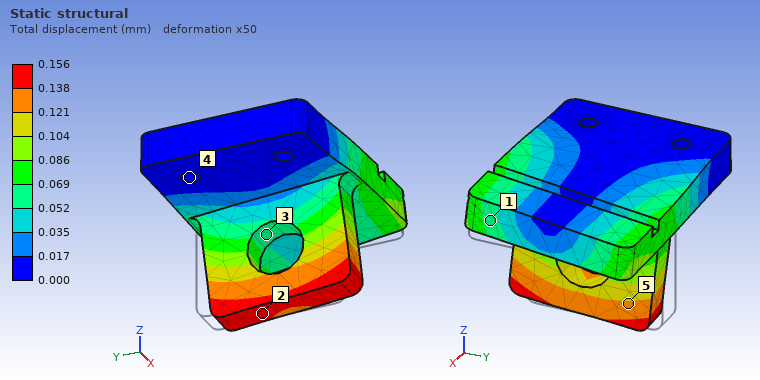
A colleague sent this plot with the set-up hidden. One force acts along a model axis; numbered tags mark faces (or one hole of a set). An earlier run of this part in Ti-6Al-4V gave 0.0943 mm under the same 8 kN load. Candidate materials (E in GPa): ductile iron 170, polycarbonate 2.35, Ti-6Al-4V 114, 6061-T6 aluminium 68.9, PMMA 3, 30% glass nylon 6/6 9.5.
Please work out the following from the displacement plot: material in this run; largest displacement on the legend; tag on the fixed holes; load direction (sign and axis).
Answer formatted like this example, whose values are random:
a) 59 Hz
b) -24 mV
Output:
a) 6061-T6 aluminium
b) 0.156 mm
c) 4
d) -Y
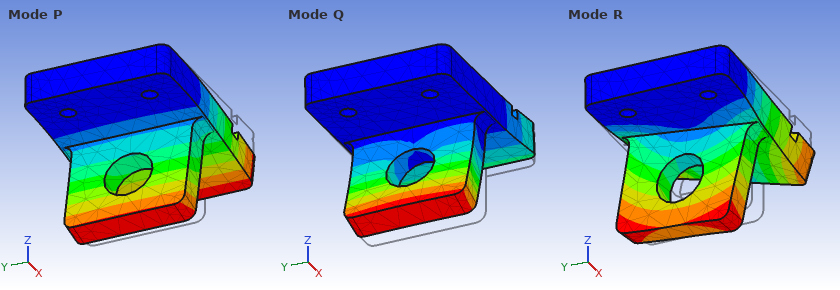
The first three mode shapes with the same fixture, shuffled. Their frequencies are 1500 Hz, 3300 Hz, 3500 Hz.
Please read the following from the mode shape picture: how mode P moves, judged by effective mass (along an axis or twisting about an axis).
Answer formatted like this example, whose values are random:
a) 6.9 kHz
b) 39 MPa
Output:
a) along Z
